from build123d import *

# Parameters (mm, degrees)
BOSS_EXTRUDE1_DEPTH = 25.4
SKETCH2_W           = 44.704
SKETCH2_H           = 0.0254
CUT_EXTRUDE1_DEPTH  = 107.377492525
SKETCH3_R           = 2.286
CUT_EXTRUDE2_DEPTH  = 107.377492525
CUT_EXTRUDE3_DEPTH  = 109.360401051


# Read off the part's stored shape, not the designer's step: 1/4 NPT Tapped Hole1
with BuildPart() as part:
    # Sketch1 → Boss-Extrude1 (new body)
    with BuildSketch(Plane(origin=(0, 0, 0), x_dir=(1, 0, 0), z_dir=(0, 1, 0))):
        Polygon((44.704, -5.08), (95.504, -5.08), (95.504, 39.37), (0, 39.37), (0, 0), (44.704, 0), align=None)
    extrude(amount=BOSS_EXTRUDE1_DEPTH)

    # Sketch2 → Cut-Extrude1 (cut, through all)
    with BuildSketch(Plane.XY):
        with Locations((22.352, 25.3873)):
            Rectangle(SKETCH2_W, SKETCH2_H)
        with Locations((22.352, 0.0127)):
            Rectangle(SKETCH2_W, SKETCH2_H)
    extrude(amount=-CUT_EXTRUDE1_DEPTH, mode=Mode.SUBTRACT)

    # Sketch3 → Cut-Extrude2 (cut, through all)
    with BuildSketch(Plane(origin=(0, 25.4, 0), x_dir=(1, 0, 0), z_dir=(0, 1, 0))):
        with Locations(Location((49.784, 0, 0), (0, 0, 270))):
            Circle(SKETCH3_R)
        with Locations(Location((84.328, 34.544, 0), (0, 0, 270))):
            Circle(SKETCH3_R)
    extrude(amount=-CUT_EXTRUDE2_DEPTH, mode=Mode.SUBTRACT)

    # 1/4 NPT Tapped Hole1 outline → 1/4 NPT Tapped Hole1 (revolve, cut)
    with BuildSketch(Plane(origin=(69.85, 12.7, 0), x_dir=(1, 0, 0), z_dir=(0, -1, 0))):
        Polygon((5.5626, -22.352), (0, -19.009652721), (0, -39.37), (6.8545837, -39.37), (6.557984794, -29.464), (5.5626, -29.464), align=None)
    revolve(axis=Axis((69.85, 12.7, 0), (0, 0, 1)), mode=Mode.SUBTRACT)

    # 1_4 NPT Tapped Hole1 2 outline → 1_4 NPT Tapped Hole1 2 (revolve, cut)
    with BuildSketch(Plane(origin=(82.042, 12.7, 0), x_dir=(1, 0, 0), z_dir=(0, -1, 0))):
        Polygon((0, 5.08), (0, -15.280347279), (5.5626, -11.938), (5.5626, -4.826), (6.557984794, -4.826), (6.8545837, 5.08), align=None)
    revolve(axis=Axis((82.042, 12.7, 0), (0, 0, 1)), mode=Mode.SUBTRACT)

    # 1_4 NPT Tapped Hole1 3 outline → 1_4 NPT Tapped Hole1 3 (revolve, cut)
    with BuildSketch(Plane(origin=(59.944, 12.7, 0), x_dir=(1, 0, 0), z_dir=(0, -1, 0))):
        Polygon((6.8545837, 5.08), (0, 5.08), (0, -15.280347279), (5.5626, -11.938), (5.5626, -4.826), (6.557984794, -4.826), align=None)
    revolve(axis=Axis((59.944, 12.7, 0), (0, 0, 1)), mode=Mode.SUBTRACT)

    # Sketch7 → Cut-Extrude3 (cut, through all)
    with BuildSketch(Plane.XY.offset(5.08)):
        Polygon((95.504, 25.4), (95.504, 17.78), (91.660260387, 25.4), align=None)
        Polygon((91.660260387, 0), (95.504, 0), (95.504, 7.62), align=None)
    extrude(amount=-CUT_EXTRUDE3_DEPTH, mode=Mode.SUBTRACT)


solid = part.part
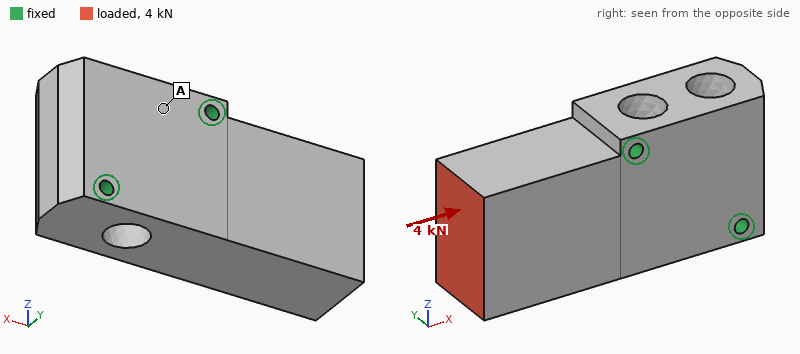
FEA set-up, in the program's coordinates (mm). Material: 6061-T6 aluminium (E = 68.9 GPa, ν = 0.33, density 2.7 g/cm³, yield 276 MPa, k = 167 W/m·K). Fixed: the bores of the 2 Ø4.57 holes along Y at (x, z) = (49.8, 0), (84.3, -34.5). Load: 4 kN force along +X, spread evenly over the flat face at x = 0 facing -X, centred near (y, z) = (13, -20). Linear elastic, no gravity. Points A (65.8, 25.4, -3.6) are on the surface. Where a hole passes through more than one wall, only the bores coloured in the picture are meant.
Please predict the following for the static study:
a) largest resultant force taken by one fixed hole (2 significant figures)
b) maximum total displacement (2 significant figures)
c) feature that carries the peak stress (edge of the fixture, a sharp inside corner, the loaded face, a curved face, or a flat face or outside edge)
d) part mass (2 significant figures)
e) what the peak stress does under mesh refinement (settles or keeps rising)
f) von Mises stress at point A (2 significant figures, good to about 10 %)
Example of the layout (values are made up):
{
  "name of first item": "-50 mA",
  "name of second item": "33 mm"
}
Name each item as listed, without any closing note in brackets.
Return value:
{
  "largest resultant force taken by one fixed hole": "2.1 kN",
  "maximum total displacement": "9.9 µm",
  "feature that carries the peak stress": "edge of the fixture",
  "part mass": "250 g",
  "what the peak stress does under mesh refinement": "keeps rising",
  "von Mises stress at point A": "2.8 MPa"
}
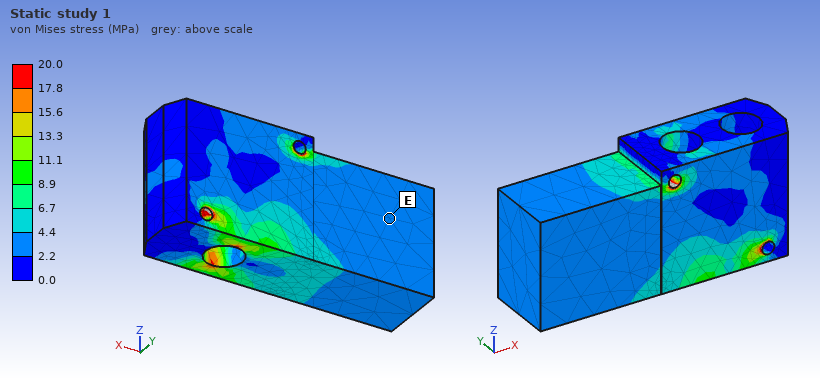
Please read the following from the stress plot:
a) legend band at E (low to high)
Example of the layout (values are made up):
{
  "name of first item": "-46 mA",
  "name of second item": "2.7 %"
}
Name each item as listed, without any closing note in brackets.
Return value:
{
  "legend band at E": "2.2 to 4.4 MPa"
}
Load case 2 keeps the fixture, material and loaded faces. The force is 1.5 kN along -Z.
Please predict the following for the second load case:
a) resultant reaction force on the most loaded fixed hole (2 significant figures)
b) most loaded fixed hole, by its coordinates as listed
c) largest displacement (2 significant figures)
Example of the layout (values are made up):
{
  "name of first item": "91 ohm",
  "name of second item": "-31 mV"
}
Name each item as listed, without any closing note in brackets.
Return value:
{
  "resultant reaction force on the most loaded fixed hole": "2.6 kN",
  "most loaded fixed hole, by its coordinates as listed": "(49.8, 0)",
  "largest displacement": "19 µm"
}
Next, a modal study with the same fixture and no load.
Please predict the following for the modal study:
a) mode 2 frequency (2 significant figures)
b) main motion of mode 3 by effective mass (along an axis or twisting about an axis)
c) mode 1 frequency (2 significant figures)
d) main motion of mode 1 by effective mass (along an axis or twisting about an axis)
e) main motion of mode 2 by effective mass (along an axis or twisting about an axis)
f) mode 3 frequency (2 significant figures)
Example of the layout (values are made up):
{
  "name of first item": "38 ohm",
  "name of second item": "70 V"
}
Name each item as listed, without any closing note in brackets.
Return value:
{
  "mode 2 frequency": "6700 Hz",
  "main motion of mode 3 by effective mass": "twisting about X",
  "mode 1 frequency": "4500 Hz",
  "main motion of mode 1 by effective mass": "along Y",
  "main motion of mode 2 by effective mass": "along Z",
  "mode 3 frequency": "9500 Hz"
}
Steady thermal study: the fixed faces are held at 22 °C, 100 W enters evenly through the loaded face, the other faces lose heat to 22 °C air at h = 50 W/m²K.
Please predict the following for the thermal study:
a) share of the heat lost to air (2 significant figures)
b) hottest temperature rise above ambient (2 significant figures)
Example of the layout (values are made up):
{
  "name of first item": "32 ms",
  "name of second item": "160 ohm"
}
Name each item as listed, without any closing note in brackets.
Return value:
{
  "share of the heat lost to air": "8.8 %",
  "hottest temperature rise above ambient": "37 K"
}
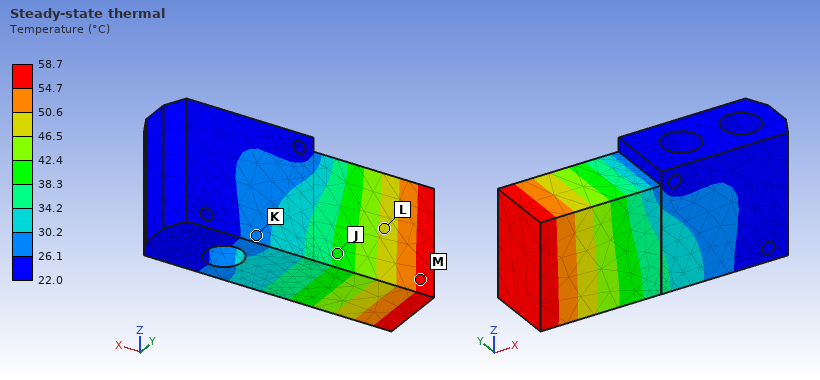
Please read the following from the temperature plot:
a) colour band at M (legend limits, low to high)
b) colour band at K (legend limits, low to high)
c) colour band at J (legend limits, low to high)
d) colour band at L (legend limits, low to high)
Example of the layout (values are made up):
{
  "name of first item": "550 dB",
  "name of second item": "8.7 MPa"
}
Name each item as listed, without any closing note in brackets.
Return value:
{
  "colour band at M": "54.7 to 58.7 °C",
  "colour band at K": "26.1 to 30.2 °C",
  "colour band at J": "38.3 to 42.4 °C",
  "colour band at L": "46.5 to 50.6 °C"
}
